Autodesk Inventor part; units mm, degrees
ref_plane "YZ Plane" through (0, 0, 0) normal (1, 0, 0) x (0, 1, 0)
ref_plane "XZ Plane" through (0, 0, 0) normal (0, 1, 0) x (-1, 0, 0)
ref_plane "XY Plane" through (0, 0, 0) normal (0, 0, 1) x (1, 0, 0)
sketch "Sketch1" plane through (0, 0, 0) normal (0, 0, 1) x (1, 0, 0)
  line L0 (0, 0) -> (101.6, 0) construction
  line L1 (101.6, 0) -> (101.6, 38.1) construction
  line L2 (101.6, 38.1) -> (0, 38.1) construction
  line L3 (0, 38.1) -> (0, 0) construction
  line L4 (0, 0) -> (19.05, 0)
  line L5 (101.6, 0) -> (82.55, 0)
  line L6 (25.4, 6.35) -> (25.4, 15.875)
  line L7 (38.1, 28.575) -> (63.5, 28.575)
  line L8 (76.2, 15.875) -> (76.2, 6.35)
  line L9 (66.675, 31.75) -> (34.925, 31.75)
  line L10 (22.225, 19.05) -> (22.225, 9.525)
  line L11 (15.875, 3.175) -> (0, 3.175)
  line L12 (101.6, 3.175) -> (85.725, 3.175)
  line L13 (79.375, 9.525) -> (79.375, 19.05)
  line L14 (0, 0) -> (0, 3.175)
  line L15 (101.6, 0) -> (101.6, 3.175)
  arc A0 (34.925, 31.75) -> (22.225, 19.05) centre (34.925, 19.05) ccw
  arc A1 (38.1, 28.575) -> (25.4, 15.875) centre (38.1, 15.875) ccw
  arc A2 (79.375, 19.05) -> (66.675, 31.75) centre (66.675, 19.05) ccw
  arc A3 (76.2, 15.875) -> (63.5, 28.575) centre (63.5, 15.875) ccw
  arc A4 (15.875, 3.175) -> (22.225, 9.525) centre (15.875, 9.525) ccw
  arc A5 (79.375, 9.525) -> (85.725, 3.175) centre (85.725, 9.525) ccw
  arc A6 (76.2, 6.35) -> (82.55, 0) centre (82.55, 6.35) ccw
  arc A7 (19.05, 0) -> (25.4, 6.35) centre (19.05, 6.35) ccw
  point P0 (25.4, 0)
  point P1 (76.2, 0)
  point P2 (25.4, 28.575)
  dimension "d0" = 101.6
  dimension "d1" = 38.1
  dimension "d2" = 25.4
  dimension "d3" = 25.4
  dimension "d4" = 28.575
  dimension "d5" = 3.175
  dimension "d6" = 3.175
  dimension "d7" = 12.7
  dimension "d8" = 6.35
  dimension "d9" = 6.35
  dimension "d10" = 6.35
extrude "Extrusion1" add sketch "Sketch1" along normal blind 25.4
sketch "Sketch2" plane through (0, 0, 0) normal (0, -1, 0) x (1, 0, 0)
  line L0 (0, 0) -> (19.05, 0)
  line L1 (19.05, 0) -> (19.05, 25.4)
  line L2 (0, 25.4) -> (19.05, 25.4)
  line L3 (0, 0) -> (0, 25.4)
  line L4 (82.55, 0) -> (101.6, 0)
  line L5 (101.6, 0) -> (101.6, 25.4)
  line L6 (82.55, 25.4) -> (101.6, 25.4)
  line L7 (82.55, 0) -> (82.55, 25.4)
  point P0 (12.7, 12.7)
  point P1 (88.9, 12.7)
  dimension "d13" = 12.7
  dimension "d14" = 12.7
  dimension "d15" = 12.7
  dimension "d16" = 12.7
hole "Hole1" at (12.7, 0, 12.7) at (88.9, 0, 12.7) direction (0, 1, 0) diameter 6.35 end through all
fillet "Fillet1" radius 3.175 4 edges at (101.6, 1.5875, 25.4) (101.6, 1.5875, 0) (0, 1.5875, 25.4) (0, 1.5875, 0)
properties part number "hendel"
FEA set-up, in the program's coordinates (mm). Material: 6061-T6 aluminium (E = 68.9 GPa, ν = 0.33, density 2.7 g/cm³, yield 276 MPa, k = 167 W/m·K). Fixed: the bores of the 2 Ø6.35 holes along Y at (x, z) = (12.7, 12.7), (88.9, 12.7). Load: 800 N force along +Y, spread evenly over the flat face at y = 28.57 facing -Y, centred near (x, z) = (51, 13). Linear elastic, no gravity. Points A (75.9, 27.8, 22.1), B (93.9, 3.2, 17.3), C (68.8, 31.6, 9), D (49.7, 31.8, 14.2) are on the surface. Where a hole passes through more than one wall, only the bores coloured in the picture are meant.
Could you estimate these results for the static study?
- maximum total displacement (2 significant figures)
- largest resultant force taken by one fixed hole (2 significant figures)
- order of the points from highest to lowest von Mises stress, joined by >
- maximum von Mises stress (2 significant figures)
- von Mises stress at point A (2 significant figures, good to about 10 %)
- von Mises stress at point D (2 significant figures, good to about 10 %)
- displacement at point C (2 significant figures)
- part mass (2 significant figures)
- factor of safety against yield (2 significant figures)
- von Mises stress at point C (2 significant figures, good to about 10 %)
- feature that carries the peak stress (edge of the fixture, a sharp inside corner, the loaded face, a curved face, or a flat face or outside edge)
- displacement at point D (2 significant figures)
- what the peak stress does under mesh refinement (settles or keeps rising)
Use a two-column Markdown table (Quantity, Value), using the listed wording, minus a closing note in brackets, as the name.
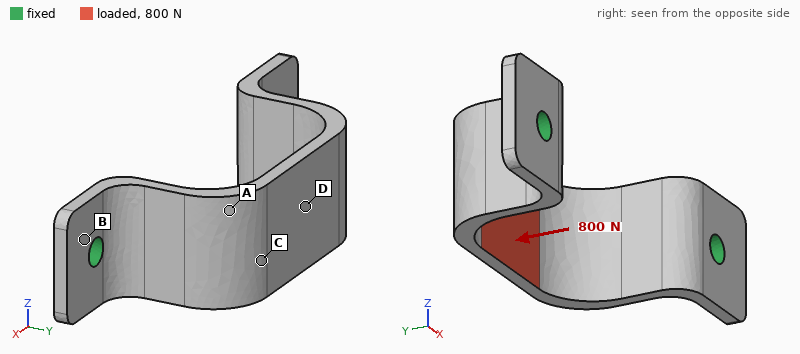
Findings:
| Quantity | Value |
|---|---|
| maximum total displacement | 85 µm |
| largest resultant force taken by one fixed hole | 510 N |
| order of the points from highest to lowest von Mises stress, joined by > | D > A > C > B |
| maximum von Mises stress | 63 MPa |
| von Mises stress at point A | 28 MPa |
| von Mises stress at point D | 56 MPa |
| displacement at point C | 24 µm |
| part mass | 34 g |
| factor of safety against yield | 4.4 |
| von Mises stress at point C | 19 MPa |
| feature that carries the peak stress | a flat face or outside edge |
| displacement at point D | 78 µm |
| what the peak stress does under mesh refinement | settles |
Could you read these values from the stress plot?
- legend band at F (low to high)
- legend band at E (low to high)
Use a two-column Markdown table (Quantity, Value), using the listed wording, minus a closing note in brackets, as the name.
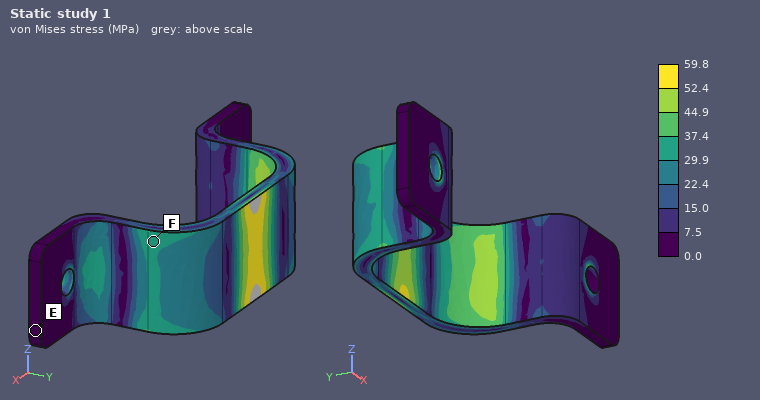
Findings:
| Quantity | Value |
|---|---|
| legend band at F | 29.9 to 37.4 MPa |
| legend band at E | 0.0 to 7.5 MPa |
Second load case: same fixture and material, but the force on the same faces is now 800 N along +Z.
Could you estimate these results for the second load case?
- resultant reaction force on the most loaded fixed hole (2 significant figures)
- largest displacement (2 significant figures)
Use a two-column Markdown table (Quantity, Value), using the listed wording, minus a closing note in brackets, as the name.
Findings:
| Quantity | Value |
|---|---|
| resultant reaction force on the most loaded fixed hole | 400 N |
| largest displacement | 0.24 mm |
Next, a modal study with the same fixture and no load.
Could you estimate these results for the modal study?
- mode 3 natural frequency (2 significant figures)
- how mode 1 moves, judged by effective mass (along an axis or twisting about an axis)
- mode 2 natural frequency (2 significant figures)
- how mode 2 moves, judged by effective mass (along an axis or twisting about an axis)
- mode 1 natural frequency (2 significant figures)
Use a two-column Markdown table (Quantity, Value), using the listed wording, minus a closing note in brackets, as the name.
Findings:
| Quantity | Value |
|---|---|
| mode 3 natural frequency | 3800 Hz |
| how mode 1 moves, judged by effective mass | along Z |
| mode 2 natural frequency | 2800 Hz |
| how mode 2 moves, judged by effective mass | along X |
| mode 1 natural frequency | 2300 Hz |
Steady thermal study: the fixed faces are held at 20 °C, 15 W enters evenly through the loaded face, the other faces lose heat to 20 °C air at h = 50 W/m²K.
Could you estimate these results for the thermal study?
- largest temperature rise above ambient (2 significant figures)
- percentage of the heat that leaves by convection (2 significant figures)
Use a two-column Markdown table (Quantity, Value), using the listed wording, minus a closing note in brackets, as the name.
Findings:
| Quantity | Value |
|---|---|
| largest temperature rise above ambient | 22 K |
| percentage of the heat that leaves by convection | 22 % |
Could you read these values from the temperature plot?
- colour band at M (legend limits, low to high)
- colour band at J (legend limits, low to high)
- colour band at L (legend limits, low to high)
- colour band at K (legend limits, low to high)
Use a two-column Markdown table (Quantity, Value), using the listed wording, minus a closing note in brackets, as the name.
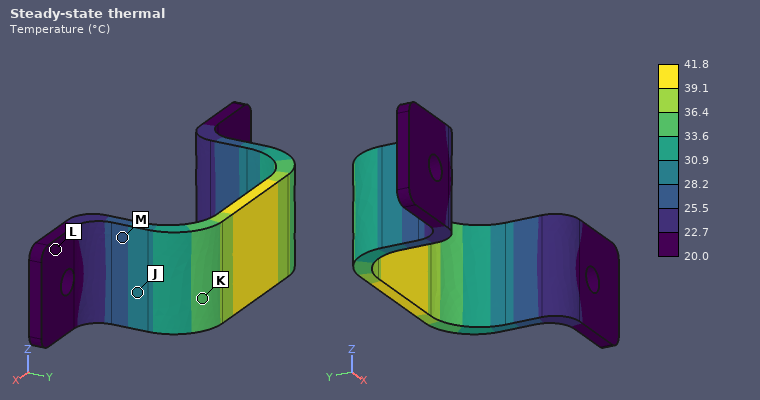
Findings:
| Quantity | Value |
|---|---|
| colour band at M | 25.5 to 28.2 °C |
| colour band at J | 28.2 to 30.9 °C |
| colour band at L | 20.0 to 22.7 °C |
| colour band at K | 33.6 to 36.4 °C |
